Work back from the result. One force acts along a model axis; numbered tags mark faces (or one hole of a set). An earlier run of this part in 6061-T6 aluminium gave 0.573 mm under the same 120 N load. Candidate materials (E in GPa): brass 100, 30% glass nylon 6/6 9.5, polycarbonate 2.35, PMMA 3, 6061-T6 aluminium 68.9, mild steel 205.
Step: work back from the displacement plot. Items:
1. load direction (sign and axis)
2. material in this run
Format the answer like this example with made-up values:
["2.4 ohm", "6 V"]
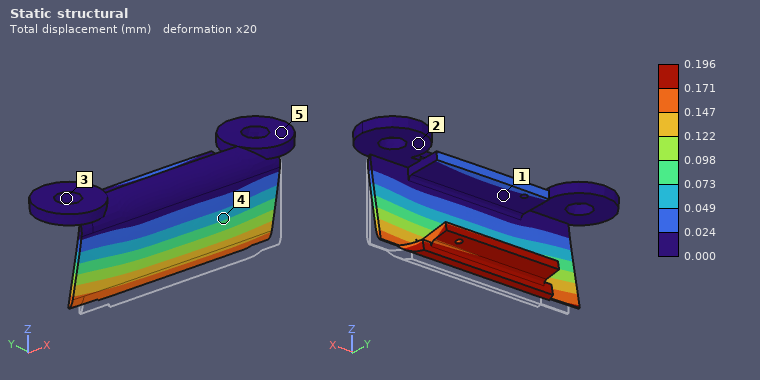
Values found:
["+Y", "mild steel"]
